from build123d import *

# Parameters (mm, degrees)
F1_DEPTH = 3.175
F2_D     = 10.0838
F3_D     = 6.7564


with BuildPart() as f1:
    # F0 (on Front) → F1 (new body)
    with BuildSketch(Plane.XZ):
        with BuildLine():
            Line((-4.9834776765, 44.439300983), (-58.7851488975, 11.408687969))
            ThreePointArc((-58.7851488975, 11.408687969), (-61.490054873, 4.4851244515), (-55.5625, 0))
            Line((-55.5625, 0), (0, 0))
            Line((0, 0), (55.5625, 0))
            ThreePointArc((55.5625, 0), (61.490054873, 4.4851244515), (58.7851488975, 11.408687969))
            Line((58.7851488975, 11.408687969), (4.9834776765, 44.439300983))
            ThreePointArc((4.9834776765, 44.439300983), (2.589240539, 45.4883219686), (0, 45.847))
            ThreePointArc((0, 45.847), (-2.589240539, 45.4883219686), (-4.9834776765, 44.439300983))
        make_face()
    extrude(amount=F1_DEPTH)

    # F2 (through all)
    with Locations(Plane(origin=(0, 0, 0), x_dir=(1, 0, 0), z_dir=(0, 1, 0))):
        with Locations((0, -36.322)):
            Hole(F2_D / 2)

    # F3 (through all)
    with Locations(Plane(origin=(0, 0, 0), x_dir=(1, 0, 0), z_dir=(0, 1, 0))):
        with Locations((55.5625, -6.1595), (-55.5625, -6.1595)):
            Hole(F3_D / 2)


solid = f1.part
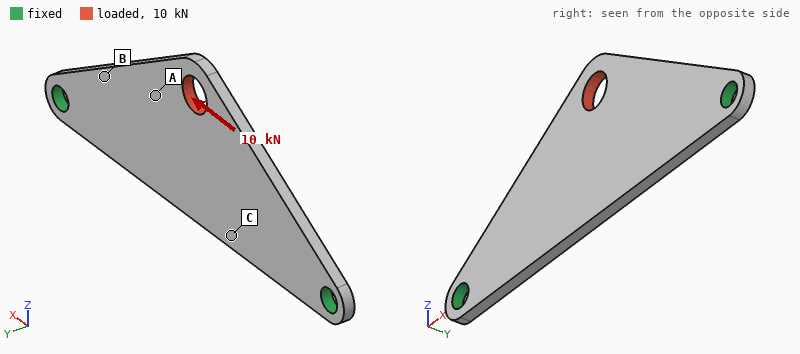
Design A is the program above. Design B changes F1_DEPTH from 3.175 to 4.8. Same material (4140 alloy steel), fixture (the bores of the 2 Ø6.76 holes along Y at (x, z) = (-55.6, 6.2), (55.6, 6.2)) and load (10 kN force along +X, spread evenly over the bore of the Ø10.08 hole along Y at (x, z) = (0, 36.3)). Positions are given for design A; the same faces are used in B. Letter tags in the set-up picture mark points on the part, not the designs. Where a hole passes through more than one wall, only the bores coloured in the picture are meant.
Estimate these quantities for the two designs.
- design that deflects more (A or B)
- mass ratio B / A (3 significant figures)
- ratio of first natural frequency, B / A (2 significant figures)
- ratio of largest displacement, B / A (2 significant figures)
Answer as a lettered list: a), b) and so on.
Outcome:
a) A
b) 1.51
c) 1.5
d) 0.66
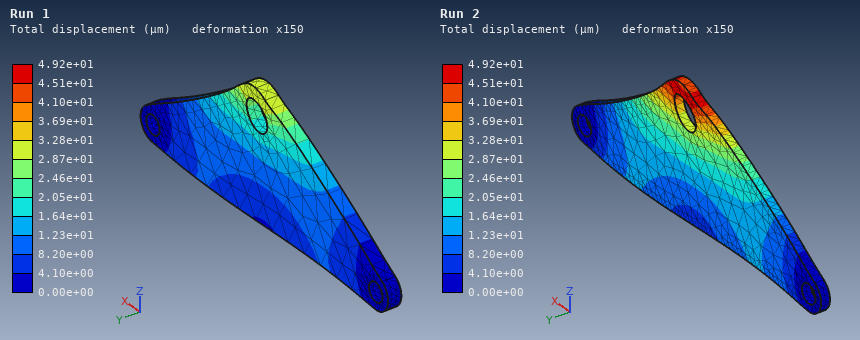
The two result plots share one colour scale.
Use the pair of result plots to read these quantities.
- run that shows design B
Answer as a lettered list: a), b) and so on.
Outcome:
a) Run 1
